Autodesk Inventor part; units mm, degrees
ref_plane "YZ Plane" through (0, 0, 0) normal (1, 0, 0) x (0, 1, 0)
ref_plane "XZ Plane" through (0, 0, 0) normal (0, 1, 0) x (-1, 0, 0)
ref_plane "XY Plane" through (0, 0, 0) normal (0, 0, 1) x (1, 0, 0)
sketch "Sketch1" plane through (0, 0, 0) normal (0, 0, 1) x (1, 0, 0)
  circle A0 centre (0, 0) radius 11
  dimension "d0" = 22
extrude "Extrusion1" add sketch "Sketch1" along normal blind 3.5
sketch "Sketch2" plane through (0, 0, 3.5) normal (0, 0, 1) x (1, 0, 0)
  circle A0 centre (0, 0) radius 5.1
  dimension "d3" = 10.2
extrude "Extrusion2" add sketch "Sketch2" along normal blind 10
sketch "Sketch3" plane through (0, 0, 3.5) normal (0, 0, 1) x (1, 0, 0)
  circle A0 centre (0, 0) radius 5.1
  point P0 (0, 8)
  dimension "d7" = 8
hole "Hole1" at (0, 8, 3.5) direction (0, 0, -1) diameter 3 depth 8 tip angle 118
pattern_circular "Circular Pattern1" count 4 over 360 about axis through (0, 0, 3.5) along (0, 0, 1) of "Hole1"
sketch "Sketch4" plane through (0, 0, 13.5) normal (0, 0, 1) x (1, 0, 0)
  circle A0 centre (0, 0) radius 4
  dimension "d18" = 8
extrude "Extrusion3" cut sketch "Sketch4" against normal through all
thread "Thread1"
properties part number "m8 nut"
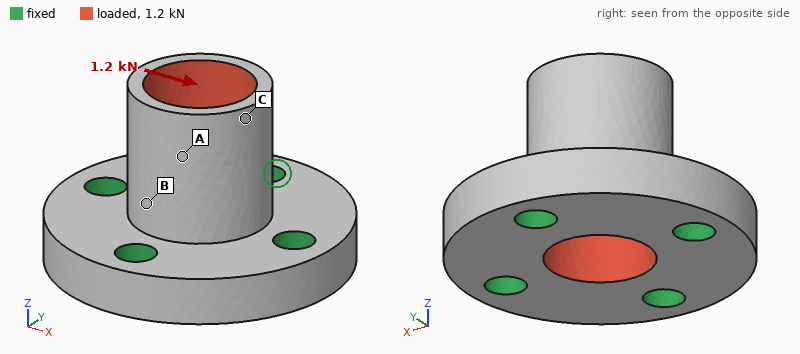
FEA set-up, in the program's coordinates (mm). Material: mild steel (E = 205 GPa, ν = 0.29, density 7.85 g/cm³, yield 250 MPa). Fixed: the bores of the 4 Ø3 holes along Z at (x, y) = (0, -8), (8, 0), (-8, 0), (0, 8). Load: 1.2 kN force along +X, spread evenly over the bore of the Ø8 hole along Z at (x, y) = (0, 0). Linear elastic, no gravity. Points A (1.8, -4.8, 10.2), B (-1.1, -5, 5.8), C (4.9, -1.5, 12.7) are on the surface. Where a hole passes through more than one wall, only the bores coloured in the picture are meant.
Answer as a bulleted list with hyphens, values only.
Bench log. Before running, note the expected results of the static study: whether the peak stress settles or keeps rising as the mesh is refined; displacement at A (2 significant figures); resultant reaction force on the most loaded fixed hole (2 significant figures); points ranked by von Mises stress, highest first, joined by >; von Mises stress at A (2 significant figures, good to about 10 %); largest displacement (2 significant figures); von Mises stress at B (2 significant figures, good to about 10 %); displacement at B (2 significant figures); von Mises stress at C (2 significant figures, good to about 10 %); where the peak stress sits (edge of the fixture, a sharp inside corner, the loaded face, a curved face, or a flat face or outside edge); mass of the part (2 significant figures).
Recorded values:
- keeps rising
- 5.7 µm
- 550 N
- B > A > C
- 29 MPa
- 8.1 µm
- 54 MPa
- 2.5 µm
- 15 MPa
- a sharp inside corner
- 11 g
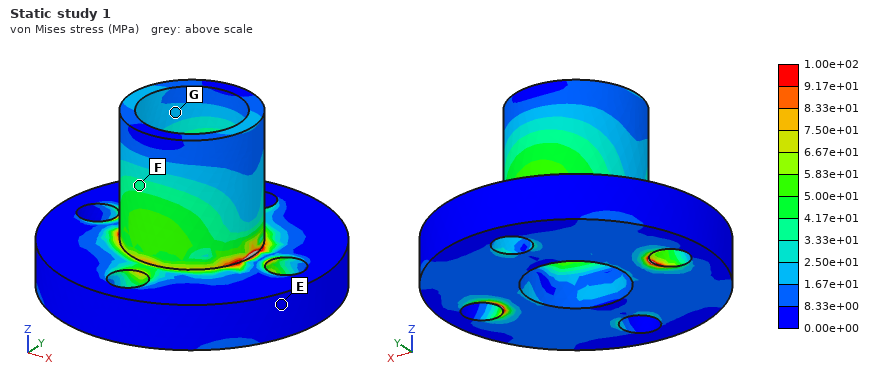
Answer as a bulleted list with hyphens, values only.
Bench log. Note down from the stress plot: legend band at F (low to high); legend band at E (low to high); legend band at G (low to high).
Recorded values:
- 3.33e+01 to 4.17e+01 MPa
- 0.00e+00 to 8.33e+00 MPa
- 1.67e+01 to 2.50e+01 MPa
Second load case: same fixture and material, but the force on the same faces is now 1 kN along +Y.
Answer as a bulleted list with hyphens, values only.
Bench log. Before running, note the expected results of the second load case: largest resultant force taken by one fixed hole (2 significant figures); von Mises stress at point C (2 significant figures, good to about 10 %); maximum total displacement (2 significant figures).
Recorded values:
- 450 N
- 6.5 MPa
- 6.8 µm
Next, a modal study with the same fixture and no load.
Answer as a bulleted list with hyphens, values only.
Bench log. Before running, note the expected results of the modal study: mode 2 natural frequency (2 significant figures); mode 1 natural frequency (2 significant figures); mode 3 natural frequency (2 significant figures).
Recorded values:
- 39 kHz
- 39 kHz
- 42 kHz
